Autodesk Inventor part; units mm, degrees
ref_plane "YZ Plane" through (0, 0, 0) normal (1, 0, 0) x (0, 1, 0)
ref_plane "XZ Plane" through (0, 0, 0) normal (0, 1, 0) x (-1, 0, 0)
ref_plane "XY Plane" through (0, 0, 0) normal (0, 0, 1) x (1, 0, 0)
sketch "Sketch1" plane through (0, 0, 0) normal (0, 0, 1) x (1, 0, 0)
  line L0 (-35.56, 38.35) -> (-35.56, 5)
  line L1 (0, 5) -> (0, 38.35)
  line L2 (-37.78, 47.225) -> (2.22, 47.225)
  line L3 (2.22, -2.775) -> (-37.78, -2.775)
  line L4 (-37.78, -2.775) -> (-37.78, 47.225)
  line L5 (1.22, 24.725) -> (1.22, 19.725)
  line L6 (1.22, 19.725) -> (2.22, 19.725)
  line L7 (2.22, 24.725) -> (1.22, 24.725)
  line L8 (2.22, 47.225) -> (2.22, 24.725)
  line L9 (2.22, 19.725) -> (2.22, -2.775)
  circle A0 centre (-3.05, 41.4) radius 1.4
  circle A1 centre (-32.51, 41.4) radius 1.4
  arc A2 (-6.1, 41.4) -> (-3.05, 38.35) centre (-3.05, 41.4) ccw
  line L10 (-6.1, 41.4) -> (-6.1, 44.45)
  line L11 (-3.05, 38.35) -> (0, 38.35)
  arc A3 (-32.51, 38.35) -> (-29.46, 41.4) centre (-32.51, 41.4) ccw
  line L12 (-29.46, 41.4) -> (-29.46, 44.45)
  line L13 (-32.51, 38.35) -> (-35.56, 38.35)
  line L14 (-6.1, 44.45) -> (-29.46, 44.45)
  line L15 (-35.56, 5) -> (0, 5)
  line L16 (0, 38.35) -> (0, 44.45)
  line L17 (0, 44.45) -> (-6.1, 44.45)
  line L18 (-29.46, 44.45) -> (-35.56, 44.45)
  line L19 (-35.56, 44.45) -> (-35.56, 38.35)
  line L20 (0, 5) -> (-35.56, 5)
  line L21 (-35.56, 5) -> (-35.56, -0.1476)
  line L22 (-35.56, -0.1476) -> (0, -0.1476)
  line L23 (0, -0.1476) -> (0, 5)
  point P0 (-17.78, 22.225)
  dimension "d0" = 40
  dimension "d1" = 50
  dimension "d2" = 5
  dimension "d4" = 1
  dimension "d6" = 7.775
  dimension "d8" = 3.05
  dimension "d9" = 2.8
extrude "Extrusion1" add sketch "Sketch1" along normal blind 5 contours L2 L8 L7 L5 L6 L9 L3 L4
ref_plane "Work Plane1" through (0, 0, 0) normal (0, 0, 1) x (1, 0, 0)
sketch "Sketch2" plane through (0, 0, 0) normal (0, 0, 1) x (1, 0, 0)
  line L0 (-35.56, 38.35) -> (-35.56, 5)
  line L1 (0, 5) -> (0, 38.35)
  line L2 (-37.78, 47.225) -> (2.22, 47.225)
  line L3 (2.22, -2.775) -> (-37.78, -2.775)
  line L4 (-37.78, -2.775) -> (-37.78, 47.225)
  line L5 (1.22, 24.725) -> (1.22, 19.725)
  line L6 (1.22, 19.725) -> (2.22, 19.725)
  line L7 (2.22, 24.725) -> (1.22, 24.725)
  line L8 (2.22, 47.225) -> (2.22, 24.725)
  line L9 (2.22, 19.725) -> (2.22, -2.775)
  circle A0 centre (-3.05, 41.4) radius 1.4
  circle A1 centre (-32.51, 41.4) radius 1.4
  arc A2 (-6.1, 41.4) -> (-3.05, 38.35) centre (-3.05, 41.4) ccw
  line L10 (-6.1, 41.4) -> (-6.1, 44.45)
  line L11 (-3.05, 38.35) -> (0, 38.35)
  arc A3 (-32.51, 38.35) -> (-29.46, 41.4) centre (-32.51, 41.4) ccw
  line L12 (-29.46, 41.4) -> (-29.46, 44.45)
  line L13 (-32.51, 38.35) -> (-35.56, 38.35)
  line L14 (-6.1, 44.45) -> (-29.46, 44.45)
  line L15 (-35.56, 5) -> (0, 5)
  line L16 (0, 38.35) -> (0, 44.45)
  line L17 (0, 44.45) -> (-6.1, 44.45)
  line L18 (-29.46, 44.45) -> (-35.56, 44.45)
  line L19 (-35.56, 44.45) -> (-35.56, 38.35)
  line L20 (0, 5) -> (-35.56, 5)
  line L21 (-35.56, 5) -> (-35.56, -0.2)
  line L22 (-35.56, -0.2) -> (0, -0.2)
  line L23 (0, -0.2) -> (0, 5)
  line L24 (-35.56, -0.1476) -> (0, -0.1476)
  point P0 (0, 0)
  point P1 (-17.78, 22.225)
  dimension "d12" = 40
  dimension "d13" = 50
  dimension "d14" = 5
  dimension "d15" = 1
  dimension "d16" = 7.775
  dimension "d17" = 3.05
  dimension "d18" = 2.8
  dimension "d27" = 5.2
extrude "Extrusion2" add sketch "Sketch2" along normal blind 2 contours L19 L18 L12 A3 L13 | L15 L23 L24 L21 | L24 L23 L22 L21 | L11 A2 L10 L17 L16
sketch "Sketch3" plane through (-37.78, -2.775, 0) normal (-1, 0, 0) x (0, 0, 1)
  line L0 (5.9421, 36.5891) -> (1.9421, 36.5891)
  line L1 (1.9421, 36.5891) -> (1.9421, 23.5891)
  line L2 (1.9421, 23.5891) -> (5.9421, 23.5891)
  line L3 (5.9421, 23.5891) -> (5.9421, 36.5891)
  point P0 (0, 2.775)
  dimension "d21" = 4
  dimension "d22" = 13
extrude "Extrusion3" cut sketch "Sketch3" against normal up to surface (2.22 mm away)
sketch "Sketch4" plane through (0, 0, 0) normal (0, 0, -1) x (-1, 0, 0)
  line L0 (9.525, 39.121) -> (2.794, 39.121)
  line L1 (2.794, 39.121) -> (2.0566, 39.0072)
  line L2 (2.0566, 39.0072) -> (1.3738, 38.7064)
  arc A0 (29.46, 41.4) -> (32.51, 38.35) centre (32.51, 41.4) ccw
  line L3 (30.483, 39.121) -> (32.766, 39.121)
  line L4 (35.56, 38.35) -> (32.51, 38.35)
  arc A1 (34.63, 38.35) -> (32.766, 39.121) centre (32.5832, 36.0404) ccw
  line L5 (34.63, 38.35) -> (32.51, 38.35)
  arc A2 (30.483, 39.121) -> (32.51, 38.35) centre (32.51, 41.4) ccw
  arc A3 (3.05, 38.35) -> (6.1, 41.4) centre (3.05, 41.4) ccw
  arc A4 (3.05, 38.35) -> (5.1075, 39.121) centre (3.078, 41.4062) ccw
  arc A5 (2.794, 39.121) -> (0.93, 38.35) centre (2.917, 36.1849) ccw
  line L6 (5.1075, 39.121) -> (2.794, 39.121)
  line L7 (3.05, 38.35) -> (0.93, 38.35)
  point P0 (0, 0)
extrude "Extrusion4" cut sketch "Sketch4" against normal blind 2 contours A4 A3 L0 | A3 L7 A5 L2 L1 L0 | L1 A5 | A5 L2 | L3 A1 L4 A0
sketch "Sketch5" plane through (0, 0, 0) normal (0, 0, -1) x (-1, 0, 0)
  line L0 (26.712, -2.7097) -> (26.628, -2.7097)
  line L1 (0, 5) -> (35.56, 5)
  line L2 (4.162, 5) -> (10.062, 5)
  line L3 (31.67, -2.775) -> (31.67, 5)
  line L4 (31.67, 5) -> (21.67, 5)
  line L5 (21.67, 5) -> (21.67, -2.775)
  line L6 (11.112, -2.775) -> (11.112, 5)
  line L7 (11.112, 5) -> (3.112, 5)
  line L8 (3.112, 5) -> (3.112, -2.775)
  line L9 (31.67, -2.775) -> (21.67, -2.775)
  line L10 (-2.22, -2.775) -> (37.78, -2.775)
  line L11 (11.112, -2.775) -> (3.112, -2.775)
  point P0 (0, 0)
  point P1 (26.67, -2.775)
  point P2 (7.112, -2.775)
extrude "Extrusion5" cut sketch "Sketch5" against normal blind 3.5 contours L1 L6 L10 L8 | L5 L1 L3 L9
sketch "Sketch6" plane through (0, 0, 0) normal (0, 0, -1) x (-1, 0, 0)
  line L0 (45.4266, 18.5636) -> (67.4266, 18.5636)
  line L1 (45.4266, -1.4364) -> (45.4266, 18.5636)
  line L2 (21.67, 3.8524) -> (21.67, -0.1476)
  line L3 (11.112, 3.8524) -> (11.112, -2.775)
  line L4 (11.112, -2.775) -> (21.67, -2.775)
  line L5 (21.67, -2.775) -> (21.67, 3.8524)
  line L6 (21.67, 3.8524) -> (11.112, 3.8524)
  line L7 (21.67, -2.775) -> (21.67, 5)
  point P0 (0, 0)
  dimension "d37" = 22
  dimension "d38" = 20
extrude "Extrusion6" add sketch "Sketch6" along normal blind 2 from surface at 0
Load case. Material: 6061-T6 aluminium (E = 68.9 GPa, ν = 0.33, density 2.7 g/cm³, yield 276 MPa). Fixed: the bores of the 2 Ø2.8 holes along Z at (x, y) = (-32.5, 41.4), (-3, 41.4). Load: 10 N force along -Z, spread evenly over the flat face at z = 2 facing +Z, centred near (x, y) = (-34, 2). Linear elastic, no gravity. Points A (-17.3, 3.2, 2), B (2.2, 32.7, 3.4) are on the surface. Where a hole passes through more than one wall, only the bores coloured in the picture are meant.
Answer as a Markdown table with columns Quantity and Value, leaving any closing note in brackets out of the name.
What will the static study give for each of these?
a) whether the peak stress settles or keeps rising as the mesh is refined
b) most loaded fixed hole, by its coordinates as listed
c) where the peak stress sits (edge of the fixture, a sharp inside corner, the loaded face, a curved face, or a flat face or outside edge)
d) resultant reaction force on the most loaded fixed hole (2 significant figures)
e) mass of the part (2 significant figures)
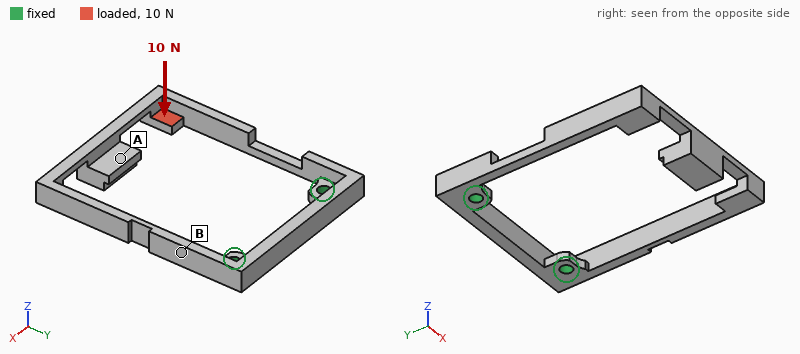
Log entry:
| Quantity | Value |
|---|---|
| whether the peak stress settles or keeps rising as the mesh is refined | keeps rising |
| most loaded fixed hole, by its coordinates as listed | (-32.5, 41.4) |
| where the peak stress sits | a sharp inside corner |
| resultant reaction force on the most loaded fixed hole | 9.2 N |
| mass of the part | 6.0 g |
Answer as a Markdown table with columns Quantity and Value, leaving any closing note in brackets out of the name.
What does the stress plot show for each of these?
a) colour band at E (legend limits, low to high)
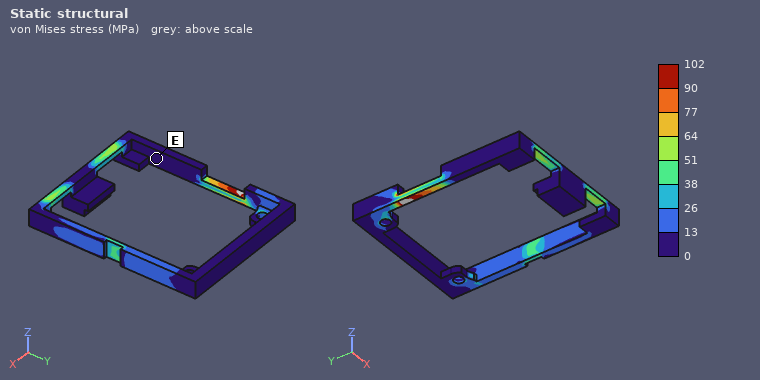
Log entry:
| Quantity | Value |
|---|---|
| colour band at E | 0 to 13 MPa |
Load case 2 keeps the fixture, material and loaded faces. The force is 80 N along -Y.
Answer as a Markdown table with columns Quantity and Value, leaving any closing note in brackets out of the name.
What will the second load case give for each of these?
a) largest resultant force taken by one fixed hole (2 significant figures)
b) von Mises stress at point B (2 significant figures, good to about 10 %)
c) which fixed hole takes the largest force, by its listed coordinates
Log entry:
| Quantity | Value |
|---|---|
| largest resultant force taken by one fixed hole | 78 N |
| von Mises stress at point B | 11 MPa |
| which fixed hole takes the largest force, by its listed coordinates | (-32.5, 41.4) |
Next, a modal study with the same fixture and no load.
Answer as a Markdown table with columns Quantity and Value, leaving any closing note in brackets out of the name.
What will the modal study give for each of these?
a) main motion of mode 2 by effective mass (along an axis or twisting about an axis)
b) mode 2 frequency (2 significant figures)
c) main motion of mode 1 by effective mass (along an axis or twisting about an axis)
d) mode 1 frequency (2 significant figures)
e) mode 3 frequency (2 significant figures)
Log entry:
| Quantity | Value |
|---|---|
| main motion of mode 2 by effective mass | along X |
| mode 2 frequency | 800 Hz |
| main motion of mode 1 by effective mass | along Z |
| mode 1 frequency | 570 Hz |
| mode 3 frequency | 1300 Hz |
